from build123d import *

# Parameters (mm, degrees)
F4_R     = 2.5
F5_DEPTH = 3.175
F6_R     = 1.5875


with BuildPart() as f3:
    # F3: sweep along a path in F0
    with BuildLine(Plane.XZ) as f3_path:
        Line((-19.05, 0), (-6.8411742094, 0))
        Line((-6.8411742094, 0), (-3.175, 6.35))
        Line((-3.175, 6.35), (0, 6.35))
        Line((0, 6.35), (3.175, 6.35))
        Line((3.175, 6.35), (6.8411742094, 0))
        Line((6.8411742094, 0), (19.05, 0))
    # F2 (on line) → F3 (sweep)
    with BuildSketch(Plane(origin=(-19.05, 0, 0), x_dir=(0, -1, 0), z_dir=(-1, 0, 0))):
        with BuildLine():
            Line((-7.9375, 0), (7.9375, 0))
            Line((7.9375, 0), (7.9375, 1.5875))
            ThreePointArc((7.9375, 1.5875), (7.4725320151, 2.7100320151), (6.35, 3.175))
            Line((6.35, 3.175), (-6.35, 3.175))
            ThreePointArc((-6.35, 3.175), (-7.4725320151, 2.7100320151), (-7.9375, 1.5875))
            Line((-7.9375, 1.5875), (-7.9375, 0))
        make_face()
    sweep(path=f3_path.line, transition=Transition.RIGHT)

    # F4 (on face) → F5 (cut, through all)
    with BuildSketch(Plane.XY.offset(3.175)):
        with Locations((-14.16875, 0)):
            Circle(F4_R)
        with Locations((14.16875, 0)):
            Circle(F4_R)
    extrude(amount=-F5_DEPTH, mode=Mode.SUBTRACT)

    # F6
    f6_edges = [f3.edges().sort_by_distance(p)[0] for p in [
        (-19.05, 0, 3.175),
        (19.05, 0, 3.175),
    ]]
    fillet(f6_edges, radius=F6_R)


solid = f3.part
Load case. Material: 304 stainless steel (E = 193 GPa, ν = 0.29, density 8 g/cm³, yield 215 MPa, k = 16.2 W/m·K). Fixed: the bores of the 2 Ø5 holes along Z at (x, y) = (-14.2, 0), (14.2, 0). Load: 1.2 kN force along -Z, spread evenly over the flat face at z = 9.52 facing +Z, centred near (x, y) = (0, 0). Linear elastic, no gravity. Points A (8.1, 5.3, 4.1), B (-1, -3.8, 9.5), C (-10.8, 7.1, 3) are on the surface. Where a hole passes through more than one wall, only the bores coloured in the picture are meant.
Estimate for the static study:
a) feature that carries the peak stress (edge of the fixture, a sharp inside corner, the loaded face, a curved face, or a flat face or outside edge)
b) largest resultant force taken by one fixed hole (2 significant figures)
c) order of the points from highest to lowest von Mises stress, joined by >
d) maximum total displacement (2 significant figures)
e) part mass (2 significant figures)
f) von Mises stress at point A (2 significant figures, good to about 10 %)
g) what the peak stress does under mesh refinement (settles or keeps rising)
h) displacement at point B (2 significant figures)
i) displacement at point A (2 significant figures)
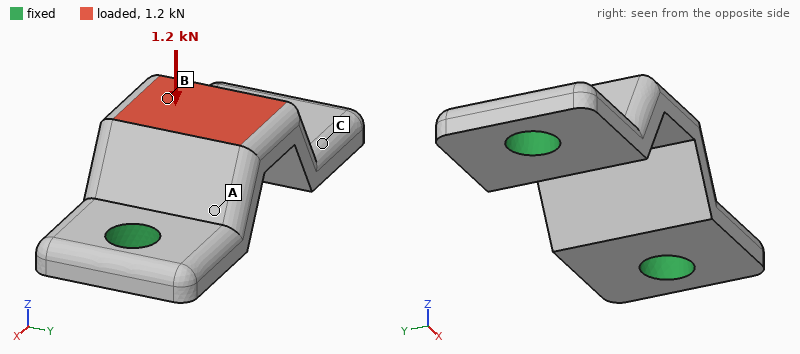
edge of the fixture
840 N
A > B > C
4.5 µm
17 g
38 MPa
keeps rising
4.4 µm
3.0 µm
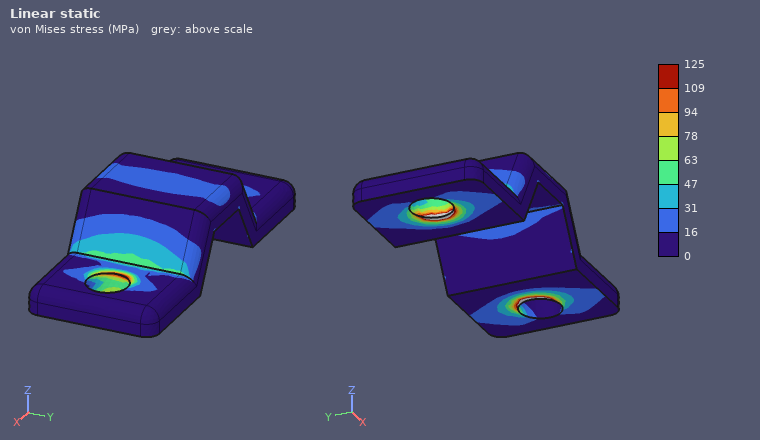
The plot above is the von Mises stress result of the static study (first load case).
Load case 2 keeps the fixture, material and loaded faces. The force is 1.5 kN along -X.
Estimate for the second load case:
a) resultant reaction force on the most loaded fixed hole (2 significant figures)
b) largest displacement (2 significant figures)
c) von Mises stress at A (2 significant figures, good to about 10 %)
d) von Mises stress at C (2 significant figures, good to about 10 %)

930 N
4.2 µm
49 MPa
16 MPa
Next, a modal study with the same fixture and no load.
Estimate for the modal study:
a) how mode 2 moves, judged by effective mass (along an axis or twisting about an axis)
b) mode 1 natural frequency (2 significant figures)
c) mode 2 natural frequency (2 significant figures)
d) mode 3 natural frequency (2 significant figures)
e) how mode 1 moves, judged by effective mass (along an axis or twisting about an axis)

along Z
16 kHz
29 kHz
37 kHz
along Y
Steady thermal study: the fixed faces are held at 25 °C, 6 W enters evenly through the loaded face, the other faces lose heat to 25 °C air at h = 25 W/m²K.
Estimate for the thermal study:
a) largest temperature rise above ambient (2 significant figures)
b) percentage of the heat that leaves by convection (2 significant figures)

53 K
12 %
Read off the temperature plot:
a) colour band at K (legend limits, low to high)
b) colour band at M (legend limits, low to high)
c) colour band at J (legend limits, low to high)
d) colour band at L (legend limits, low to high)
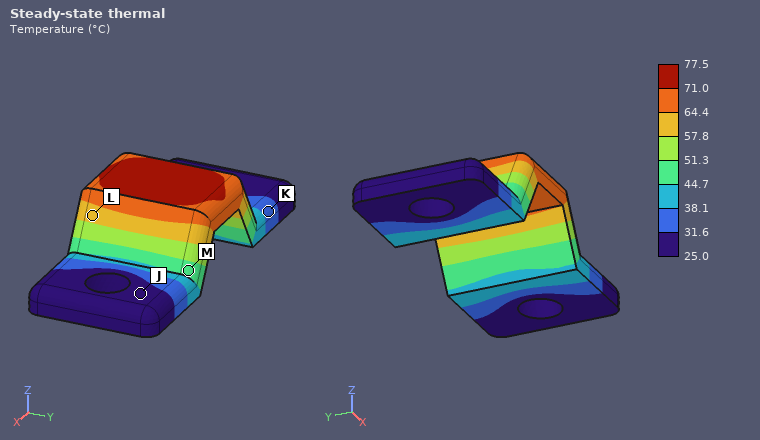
31.6 to 38.1 °C
44.7 to 51.3 °C
25.0 to 31.6 °C
57.8 to 64.4 °C
